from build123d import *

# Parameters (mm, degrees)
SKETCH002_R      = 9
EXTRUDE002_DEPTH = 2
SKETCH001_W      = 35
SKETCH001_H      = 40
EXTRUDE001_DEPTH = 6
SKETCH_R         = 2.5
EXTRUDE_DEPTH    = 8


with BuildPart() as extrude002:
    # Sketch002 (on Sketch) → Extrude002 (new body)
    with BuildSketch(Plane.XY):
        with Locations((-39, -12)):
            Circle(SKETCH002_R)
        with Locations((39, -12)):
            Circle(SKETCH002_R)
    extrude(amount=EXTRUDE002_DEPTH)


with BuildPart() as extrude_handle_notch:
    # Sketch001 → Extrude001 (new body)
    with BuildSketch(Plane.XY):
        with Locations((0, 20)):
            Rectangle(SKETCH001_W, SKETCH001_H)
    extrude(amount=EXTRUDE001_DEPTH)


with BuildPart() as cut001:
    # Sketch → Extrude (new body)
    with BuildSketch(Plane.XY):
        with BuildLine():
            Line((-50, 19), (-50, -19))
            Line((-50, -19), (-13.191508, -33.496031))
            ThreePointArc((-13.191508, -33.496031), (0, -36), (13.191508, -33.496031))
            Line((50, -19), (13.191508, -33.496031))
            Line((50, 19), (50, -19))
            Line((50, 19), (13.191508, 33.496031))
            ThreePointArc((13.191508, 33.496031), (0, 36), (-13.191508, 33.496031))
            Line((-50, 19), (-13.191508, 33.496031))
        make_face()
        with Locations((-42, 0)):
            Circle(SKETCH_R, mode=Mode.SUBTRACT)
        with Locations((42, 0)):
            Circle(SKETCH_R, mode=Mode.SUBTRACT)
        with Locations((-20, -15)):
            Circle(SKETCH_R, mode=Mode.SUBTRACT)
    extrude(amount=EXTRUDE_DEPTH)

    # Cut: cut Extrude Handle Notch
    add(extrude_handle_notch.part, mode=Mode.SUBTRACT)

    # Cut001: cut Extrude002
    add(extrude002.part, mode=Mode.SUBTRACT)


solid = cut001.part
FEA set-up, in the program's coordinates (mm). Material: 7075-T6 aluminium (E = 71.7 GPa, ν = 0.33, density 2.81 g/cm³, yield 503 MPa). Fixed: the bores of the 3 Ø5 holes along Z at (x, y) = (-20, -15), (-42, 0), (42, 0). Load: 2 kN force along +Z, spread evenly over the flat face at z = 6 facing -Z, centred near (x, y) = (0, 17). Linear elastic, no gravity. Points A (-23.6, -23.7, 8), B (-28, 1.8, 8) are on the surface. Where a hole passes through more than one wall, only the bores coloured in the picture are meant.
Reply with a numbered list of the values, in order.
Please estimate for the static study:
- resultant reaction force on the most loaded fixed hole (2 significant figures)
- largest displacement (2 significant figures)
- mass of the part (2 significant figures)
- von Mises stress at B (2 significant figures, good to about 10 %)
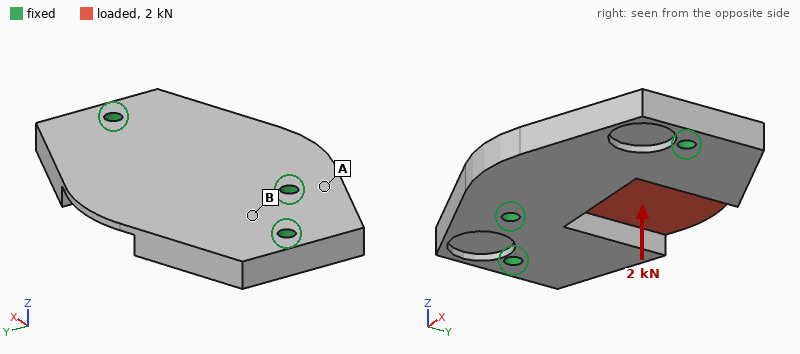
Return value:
1. 1.3 kN
2. 0.43 mm
3. 100 g
4. 41 MPa
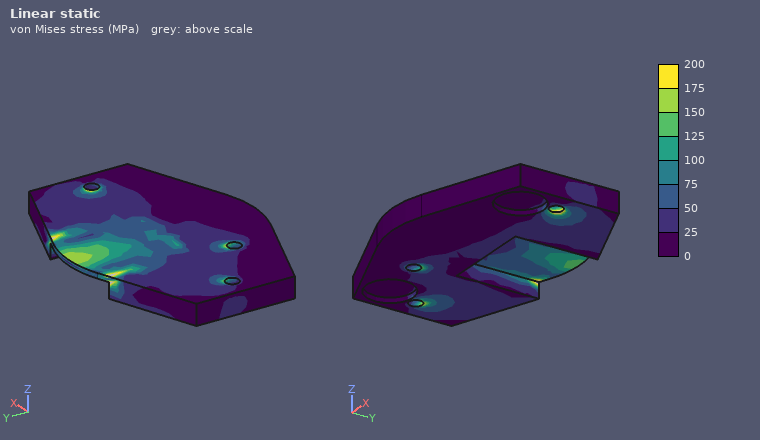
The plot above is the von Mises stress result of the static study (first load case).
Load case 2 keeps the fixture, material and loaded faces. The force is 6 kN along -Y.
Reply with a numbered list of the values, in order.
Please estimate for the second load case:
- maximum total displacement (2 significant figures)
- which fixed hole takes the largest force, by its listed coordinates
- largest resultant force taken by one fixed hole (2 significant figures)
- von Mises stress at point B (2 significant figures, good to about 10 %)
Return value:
1. 59 µm
2. (-20, -15)
3. 3.5 kN
4. 16 MPa
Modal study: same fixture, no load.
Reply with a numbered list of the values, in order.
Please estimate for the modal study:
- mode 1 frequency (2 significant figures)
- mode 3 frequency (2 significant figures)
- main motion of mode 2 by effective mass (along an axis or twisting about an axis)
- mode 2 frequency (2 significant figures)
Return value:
1. 4600 Hz
2. 6500 Hz
3. along Z
4. 6100 Hz
